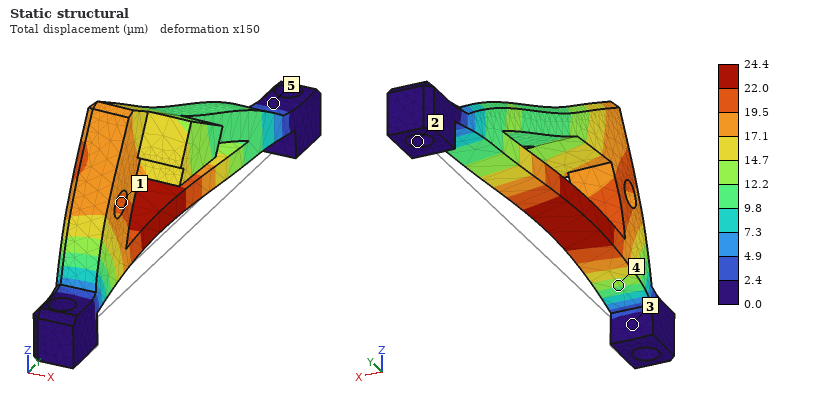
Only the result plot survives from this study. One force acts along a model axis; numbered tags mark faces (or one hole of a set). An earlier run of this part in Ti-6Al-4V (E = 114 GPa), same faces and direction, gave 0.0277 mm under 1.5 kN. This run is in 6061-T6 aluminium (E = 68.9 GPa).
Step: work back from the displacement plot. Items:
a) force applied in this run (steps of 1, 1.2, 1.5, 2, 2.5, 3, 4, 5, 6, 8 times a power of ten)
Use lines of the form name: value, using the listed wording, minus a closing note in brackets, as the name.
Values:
force applied in this run: 800 N
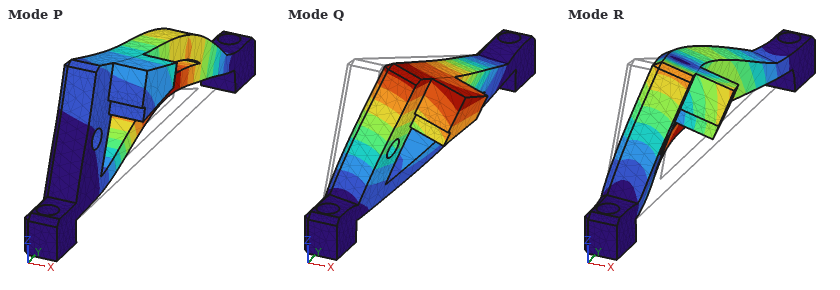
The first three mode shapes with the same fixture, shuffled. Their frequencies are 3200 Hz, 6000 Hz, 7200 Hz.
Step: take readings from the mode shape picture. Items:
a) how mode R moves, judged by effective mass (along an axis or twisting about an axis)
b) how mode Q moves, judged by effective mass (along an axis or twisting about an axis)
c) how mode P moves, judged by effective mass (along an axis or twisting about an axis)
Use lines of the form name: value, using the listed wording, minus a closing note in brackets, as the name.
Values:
how mode R moves, judged by effective mass: along X
how mode Q moves, judged by effective mass: along X
how mode P moves, judged by effective mass: along Z
